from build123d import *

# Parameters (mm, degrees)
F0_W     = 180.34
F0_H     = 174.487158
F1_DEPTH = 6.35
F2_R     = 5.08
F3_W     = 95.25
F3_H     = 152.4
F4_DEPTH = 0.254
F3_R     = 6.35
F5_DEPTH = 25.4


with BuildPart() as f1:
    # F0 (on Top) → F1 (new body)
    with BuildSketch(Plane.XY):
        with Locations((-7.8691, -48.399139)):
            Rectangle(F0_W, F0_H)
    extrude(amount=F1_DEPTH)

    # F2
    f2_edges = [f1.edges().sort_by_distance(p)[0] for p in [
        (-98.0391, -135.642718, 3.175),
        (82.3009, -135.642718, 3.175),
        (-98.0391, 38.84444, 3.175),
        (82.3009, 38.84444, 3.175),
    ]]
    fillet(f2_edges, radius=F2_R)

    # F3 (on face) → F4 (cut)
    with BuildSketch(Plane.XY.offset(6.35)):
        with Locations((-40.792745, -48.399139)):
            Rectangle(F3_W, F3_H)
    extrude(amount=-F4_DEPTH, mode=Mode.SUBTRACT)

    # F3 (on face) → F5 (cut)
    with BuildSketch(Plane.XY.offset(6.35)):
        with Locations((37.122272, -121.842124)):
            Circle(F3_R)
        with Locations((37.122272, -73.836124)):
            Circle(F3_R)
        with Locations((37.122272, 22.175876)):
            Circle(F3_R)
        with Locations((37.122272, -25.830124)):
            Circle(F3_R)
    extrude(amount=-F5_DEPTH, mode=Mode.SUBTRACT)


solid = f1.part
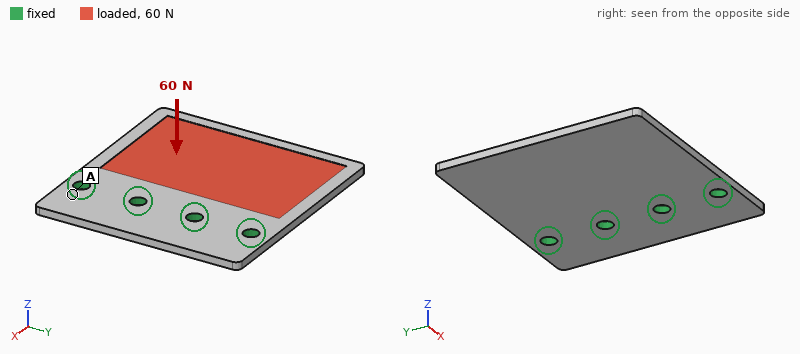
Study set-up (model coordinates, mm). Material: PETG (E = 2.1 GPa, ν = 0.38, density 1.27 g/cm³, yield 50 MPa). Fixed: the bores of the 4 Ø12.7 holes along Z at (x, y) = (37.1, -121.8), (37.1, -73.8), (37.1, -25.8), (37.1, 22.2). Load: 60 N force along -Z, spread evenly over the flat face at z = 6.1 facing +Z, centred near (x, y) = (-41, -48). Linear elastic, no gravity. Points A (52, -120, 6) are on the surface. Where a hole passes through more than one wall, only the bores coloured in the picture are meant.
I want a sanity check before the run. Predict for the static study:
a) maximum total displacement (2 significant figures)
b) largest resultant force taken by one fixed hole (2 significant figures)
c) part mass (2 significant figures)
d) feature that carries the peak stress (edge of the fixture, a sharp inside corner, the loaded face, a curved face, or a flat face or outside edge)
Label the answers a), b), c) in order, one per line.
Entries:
a) 2.4 mm
b) 22 N
c) 240 g
d) a flat face or outside edge
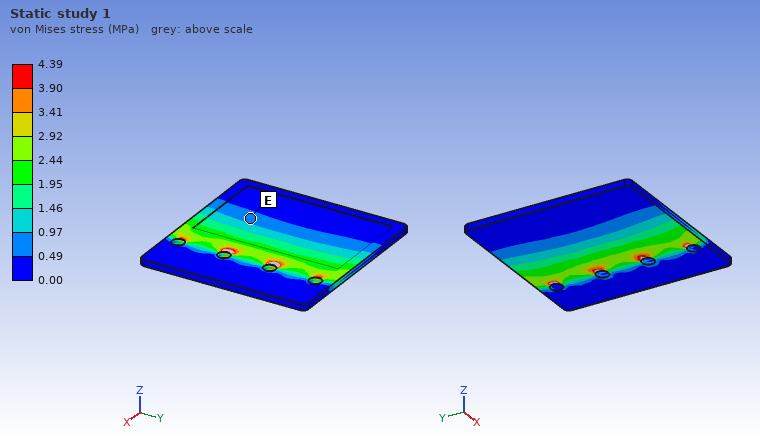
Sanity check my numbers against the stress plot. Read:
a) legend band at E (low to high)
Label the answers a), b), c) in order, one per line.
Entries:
a) 0.49 to 0.97 MPa
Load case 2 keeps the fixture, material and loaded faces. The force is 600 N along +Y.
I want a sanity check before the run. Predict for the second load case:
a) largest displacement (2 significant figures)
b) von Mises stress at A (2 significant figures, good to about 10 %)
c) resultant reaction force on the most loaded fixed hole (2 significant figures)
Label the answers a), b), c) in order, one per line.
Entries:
a) 0.63 mm
b) 0.28 MPa
c) 320 N
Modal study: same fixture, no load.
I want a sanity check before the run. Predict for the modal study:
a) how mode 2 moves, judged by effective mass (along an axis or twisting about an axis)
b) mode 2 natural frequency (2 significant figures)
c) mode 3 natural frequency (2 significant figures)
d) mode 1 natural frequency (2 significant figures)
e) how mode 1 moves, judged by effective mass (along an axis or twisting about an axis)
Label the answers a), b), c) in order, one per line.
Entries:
a) twisting about X
b) 150 Hz
c) 370 Hz
d) 79 Hz
e) along Z
